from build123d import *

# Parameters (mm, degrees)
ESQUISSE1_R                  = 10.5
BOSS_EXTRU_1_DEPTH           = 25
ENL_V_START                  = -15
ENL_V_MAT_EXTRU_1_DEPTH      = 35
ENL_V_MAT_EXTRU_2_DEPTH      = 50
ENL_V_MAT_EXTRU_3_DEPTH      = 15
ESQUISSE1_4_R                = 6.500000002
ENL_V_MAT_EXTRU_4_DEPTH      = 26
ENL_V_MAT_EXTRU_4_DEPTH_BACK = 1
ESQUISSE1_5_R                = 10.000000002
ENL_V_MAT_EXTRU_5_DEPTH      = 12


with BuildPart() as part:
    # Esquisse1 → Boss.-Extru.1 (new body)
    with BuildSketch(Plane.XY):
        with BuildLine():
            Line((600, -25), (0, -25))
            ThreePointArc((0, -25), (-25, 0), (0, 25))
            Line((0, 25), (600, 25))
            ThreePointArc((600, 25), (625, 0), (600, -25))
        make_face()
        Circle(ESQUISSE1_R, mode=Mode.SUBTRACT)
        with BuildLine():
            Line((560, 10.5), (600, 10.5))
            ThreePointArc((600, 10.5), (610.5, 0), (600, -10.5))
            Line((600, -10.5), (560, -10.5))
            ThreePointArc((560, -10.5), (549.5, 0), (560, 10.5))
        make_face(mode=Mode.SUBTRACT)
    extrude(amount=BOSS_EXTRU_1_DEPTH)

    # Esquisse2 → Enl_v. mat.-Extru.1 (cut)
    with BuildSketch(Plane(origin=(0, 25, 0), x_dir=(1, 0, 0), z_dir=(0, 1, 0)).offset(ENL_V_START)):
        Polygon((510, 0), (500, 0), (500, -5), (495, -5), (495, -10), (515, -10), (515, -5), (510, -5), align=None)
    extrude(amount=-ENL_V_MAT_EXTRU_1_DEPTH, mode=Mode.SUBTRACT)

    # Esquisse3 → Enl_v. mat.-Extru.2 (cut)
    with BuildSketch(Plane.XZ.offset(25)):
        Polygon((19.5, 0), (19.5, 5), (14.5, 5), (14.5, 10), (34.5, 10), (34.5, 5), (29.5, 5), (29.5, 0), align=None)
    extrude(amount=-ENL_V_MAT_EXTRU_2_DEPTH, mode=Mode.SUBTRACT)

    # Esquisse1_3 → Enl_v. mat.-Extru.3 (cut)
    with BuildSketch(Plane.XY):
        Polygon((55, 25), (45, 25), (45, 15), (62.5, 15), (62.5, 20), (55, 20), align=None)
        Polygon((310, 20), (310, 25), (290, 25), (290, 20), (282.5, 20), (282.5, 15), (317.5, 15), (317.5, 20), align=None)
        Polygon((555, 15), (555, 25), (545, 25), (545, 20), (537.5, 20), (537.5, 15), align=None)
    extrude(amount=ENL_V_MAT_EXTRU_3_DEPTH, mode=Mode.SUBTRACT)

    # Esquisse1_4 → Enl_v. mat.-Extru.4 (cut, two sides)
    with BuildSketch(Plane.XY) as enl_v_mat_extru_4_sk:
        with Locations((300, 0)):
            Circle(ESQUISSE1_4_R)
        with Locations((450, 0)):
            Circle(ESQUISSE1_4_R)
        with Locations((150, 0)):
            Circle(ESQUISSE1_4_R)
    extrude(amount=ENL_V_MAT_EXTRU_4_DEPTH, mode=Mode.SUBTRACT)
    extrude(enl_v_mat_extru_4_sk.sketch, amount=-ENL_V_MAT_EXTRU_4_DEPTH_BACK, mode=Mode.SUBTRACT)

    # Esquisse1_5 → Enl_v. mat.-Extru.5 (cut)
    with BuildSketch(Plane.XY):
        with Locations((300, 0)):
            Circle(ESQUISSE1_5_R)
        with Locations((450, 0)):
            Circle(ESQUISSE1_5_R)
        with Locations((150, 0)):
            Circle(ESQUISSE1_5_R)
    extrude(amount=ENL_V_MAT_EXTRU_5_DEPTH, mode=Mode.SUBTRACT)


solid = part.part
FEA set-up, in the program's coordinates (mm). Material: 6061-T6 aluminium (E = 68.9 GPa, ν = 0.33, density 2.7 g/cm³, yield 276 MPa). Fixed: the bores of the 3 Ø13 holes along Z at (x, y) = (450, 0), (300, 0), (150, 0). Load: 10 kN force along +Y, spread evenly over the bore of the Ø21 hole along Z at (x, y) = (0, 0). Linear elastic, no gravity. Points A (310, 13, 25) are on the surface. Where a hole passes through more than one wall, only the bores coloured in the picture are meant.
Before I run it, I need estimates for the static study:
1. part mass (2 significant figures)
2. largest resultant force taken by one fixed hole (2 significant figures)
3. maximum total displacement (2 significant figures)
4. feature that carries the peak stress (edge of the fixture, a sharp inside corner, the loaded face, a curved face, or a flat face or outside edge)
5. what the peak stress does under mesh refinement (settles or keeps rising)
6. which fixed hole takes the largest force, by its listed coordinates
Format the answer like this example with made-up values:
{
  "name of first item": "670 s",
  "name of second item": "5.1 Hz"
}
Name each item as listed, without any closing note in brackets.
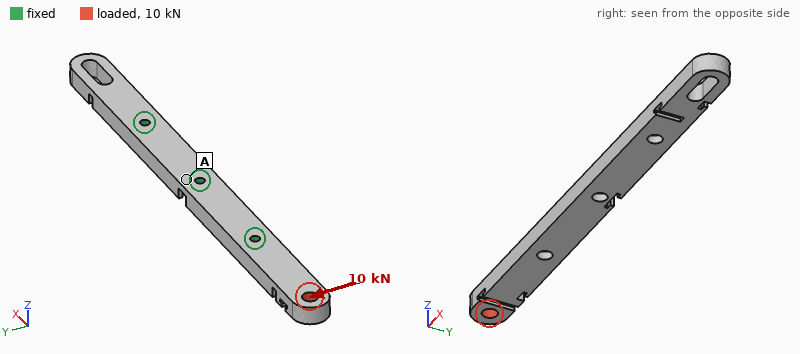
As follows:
{
  "part mass": "2.0 kg",
  "largest resultant force taken by one fixed hole": "18 kN",
  "maximum total displacement": "1.4 mm",
  "feature that carries the peak stress": "edge of the fixture",
  "what the peak stress does under mesh refinement": "keeps rising",
  "which fixed hole takes the largest force, by its listed coordinates": "(150, 0)"
}
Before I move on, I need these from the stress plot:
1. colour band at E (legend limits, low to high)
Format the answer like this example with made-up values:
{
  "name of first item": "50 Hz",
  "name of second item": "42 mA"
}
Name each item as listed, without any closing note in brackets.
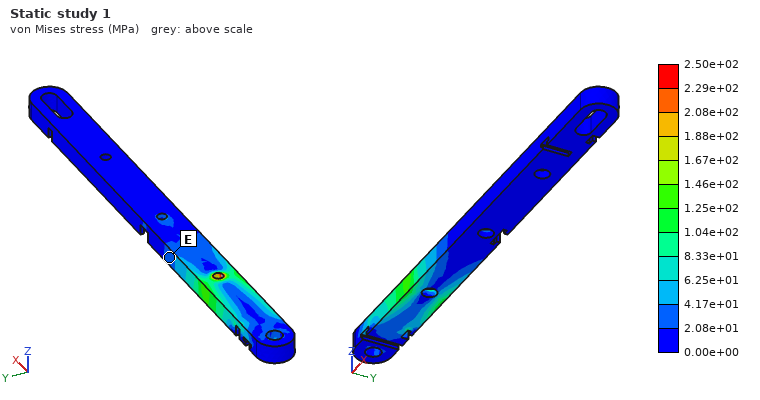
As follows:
{
  "colour band at E": "2.08e+01 to 4.17e+01 MPa"
}
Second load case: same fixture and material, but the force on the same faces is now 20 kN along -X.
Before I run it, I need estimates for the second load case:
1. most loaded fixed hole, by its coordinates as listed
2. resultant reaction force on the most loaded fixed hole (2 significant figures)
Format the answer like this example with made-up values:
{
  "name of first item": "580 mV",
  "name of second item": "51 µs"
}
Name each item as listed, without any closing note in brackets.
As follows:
{
  "most loaded fixed hole, by its coordinates as listed": "(150, 0)",
  "resultant reaction force on the most loaded fixed hole": "17 kN"
}
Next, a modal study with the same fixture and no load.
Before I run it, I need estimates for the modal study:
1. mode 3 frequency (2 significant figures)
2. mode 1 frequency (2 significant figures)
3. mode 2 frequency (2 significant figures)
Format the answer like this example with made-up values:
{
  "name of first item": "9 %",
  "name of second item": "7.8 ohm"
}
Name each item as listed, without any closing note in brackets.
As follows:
{
  "mode 3 frequency": "1100 Hz",
  "mode 1 frequency": "620 Hz",
  "mode 2 frequency": "640 Hz"
}
